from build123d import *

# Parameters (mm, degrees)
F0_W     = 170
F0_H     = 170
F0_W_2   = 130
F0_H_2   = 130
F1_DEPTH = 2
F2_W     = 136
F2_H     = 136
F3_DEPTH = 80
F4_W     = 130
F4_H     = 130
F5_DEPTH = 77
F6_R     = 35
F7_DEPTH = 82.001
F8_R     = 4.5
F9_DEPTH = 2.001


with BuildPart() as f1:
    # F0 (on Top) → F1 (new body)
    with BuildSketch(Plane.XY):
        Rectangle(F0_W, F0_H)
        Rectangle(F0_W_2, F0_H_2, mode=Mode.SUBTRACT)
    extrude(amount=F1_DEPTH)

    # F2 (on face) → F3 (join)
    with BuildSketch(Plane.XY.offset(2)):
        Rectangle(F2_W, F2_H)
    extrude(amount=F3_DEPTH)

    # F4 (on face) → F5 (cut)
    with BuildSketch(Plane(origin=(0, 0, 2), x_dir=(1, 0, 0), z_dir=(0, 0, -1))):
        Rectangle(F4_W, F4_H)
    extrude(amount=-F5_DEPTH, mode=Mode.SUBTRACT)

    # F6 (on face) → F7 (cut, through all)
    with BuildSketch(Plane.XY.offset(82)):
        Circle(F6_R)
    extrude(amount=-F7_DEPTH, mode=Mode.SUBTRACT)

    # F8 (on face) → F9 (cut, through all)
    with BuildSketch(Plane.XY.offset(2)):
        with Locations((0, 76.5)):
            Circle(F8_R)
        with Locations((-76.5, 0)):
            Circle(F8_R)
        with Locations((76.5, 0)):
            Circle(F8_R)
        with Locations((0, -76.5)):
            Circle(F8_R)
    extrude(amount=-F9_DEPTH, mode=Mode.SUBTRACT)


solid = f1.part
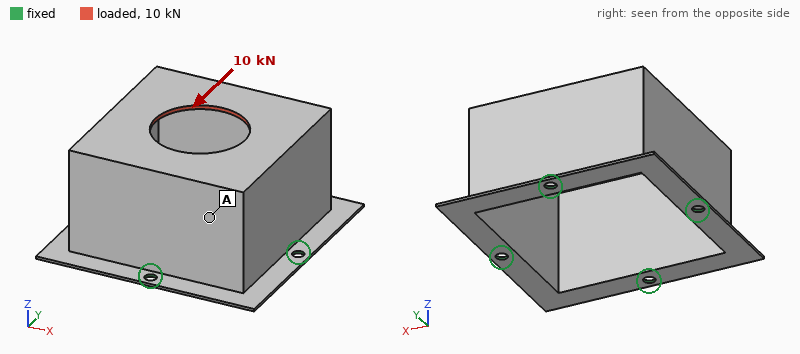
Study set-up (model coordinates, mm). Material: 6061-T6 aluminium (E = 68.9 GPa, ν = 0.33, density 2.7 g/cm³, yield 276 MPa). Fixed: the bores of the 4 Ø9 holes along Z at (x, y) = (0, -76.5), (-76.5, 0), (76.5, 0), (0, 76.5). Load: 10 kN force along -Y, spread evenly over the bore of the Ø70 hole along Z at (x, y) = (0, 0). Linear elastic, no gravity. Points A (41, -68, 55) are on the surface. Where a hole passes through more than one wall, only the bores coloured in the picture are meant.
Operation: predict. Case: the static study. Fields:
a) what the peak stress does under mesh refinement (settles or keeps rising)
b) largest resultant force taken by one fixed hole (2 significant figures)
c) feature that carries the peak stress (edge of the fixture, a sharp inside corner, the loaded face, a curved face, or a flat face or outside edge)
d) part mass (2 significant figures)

keeps rising
5.8 kN
edge of the fixture
510 g
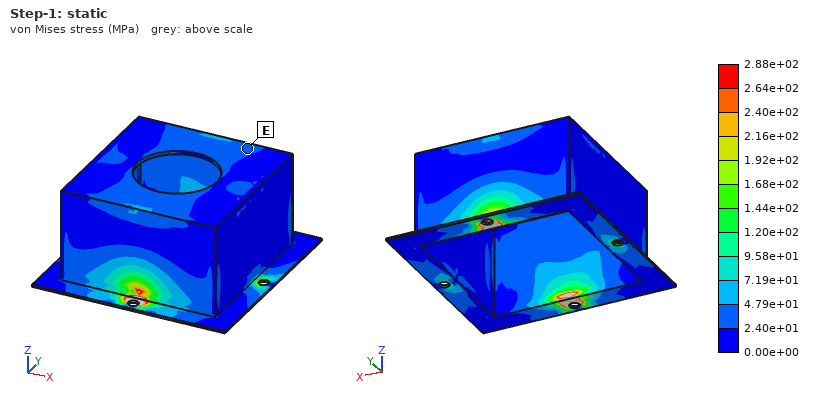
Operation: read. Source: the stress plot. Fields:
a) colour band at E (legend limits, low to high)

2.40e+01 to 4.79e+01 MPa
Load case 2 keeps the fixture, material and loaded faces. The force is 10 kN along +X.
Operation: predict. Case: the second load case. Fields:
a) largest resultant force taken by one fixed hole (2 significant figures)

5.8 kN
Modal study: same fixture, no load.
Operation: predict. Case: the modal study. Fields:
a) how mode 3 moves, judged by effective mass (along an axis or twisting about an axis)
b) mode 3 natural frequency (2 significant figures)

along Z
1500 Hz
